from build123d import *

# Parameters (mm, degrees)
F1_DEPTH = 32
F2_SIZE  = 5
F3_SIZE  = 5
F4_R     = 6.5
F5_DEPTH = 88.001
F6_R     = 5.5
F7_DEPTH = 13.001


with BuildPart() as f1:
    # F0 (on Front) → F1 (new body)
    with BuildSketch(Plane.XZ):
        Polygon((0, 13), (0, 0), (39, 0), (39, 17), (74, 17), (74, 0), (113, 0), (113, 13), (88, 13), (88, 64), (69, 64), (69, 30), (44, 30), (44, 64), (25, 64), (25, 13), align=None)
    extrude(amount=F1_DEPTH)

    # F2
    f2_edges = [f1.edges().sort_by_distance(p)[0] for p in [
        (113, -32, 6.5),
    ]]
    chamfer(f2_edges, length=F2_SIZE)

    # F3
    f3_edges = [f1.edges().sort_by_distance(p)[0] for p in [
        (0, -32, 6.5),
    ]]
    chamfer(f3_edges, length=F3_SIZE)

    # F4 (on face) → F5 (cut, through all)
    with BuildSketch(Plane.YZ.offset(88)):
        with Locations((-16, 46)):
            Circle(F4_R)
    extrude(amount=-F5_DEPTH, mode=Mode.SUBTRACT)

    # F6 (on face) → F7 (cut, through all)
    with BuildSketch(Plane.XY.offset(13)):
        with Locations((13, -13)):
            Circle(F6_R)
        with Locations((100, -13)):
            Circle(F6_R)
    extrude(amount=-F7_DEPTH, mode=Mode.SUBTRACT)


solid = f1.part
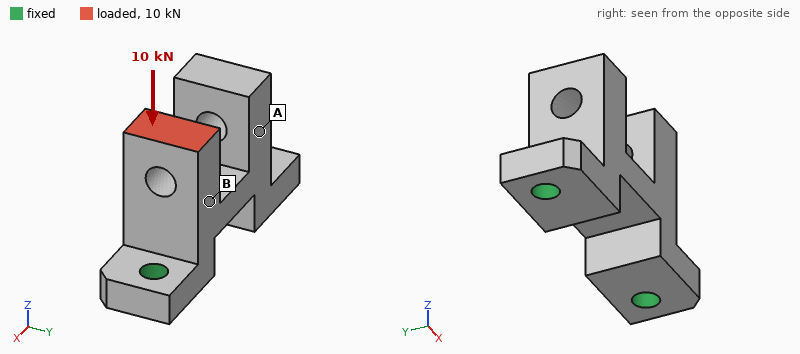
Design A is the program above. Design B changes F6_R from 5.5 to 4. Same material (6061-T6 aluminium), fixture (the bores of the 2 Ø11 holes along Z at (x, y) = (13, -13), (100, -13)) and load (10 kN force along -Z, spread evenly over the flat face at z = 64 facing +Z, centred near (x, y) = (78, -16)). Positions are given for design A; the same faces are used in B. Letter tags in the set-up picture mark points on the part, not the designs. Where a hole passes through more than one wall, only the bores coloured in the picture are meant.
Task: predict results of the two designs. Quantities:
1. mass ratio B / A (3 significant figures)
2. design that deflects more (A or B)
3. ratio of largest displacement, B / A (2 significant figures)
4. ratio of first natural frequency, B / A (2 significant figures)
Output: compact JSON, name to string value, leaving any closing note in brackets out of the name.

{"mass ratio B / A": "1.01", "design that deflects more": "B", "ratio of largest displacement, B / A": "1.2", "ratio of first natural frequency, B / A": "0.90"}
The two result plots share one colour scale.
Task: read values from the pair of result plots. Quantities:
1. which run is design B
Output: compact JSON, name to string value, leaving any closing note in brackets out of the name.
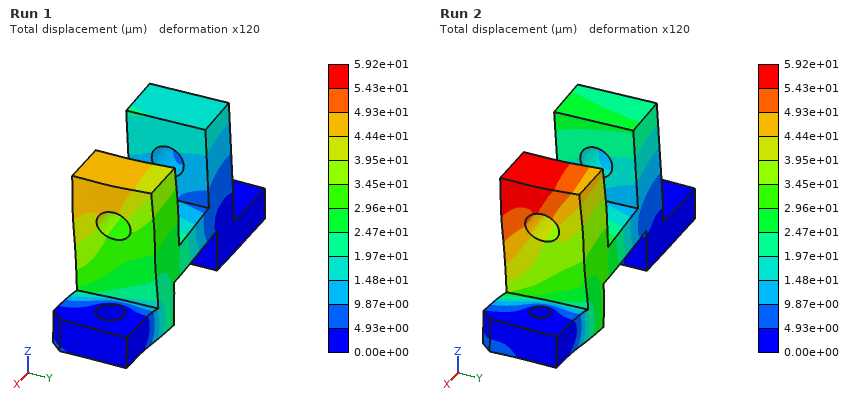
{"which run is design B": "Run 2"}
